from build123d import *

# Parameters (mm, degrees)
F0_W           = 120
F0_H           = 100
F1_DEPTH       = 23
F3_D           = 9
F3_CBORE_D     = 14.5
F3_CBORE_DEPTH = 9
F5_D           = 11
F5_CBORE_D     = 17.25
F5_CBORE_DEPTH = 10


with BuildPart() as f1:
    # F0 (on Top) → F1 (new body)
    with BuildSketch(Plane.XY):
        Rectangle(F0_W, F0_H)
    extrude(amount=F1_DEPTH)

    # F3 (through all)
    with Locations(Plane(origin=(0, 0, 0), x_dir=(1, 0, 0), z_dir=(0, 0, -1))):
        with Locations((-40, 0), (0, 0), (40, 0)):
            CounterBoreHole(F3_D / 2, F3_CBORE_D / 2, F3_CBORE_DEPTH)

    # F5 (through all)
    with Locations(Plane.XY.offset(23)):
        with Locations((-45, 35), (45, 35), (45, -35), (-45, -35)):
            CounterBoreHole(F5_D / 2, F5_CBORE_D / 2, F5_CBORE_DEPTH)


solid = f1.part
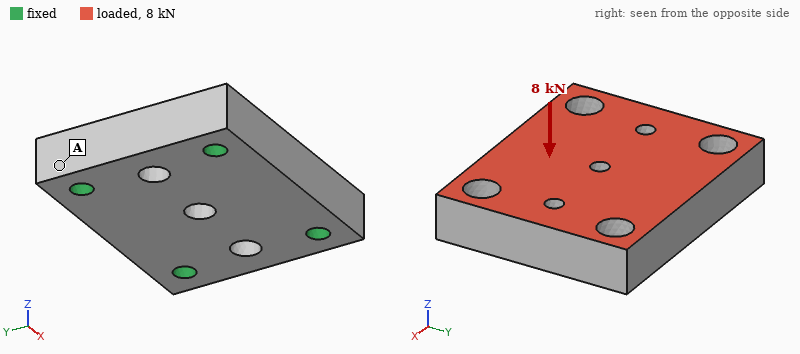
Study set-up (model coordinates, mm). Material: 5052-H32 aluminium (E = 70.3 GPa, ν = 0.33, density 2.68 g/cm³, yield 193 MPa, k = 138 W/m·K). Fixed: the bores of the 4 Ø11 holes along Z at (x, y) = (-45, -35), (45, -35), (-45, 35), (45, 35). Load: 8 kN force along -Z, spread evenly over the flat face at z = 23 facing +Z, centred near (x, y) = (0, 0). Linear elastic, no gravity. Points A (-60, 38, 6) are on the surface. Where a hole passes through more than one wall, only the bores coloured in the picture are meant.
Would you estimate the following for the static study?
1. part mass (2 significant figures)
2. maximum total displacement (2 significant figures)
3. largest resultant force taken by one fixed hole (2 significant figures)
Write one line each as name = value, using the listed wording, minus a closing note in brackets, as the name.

part mass = 680 g
maximum total displacement = 6.2 µm
largest resultant force taken by one fixed hole = 2.2 kN
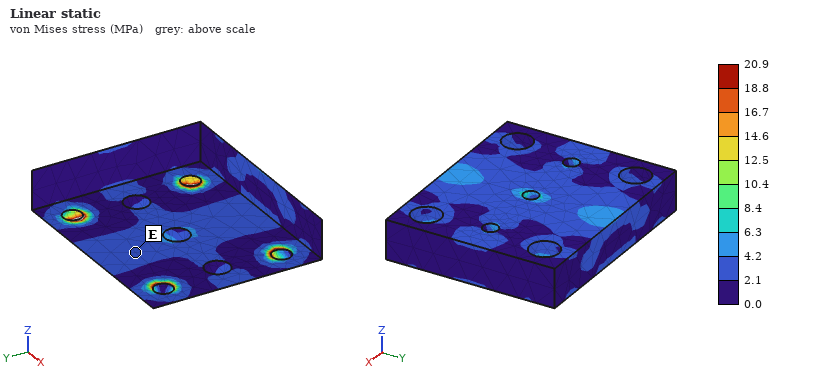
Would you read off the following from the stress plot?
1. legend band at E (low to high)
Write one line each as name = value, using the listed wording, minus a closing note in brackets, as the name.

legend band at E = 2.1 to 4.2 MPa
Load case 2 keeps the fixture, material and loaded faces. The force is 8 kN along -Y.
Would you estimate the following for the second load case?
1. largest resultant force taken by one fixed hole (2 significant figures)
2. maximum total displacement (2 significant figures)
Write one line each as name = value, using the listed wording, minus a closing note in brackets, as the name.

largest resultant force taken by one fixed hole = 2.2 kN
maximum total displacement = 4.5 µm
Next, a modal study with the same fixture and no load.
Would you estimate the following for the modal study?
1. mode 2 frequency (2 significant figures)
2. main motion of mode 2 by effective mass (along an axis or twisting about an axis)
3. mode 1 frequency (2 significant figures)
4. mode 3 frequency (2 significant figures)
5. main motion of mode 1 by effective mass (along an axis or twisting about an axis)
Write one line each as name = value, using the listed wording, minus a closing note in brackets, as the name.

mode 2 frequency = 11 kHz
main motion of mode 2 by effective mass = twisting about X
mode 1 frequency = 8100 Hz
mode 3 frequency = 13 kHz
main motion of mode 1 by effective mass = along Z
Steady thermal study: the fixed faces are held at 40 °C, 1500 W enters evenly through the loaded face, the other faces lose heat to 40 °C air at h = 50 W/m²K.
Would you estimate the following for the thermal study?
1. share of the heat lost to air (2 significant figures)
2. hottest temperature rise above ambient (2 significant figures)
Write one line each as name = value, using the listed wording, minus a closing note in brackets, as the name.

share of the heat lost to air = 3.9 %
hottest temperature rise above ambient = 82 K
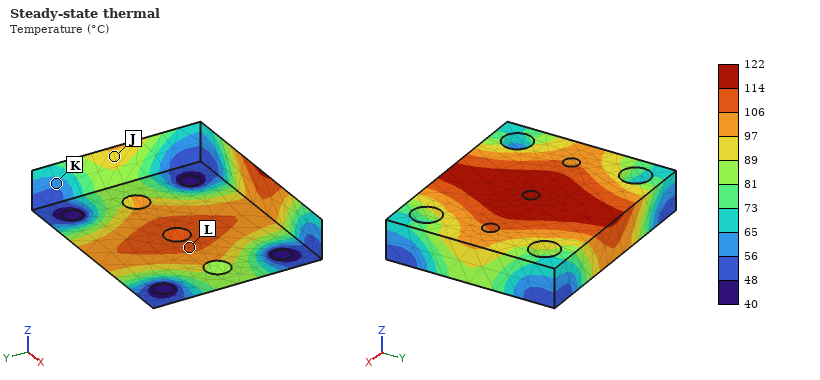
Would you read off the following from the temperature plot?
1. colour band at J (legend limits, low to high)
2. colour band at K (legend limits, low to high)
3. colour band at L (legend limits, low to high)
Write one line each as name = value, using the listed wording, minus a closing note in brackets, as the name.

colour band at J = 89 to 97 °C
colour band at K = 56 to 65 °C
colour band at L = 106 to 114 °C
